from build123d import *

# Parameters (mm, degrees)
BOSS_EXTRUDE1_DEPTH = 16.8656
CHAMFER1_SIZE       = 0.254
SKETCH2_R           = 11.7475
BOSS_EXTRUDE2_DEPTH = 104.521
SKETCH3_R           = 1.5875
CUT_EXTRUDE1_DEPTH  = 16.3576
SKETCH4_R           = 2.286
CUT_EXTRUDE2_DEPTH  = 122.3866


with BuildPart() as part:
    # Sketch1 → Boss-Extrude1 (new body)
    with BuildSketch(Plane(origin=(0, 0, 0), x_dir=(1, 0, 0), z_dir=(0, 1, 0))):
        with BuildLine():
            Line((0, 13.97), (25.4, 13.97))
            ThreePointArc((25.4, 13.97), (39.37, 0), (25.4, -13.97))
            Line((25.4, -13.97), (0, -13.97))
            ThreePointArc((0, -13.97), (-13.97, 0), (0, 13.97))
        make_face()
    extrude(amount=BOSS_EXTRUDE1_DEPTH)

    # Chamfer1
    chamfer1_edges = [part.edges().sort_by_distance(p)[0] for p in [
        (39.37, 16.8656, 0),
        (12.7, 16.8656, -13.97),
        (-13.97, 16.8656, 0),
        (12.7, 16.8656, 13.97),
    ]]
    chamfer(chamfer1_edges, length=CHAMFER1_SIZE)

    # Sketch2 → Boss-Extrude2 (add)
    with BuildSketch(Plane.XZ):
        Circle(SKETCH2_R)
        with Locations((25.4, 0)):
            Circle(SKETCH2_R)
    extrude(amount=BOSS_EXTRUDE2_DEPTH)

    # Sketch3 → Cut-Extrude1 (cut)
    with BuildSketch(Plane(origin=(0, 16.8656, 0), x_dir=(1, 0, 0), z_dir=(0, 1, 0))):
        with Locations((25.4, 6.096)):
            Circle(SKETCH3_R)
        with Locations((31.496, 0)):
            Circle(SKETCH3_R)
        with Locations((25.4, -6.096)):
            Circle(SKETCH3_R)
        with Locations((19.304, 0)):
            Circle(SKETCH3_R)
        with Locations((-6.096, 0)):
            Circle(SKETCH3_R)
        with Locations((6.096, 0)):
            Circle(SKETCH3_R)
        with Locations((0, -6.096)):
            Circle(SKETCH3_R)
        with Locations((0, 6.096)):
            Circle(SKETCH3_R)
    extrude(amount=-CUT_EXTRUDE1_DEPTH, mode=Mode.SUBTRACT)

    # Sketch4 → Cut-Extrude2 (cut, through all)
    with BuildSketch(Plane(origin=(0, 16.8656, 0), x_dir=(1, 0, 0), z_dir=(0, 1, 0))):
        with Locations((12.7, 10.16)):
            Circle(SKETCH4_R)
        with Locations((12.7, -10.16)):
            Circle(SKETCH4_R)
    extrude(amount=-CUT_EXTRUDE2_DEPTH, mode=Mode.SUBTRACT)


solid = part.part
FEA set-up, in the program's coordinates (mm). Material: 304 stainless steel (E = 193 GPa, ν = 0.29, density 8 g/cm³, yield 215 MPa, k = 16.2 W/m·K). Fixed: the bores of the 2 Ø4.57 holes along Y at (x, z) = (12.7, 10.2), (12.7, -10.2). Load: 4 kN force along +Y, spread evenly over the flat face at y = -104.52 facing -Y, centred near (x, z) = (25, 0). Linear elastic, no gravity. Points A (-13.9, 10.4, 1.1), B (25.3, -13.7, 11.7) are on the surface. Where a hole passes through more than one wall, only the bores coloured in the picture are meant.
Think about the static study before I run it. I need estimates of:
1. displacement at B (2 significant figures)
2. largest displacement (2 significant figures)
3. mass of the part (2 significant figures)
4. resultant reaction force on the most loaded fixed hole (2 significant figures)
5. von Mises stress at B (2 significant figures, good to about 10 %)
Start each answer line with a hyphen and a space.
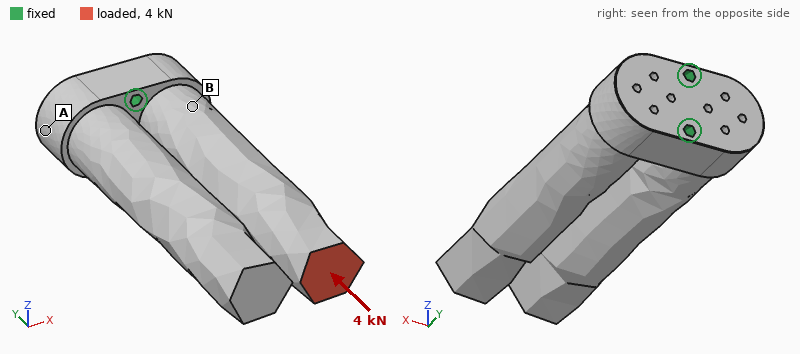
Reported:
- 5.9 µm
- 27 µm
- 890 g
- 2.0 kN
- 8.6 MPa
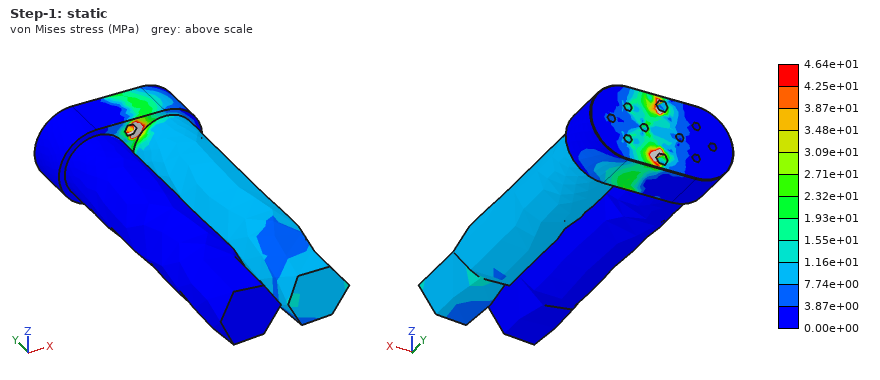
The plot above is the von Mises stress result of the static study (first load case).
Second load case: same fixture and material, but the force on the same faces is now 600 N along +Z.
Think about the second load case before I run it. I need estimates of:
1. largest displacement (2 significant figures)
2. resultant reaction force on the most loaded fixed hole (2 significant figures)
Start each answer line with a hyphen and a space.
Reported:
- 0.11 mm
- 2.7 kN
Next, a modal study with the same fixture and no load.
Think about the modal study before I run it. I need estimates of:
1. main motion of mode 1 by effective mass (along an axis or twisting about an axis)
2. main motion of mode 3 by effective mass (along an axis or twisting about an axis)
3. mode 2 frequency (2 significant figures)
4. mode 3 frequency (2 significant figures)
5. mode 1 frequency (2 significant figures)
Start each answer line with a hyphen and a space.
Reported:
- along X
- along Z
- 1100 Hz
- 1200 Hz
- 1000 Hz
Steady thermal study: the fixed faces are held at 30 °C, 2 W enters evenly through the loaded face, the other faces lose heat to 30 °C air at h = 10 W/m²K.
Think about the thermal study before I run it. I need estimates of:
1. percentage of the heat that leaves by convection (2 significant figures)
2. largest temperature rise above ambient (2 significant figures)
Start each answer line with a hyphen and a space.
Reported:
- 47 %
- 23 K
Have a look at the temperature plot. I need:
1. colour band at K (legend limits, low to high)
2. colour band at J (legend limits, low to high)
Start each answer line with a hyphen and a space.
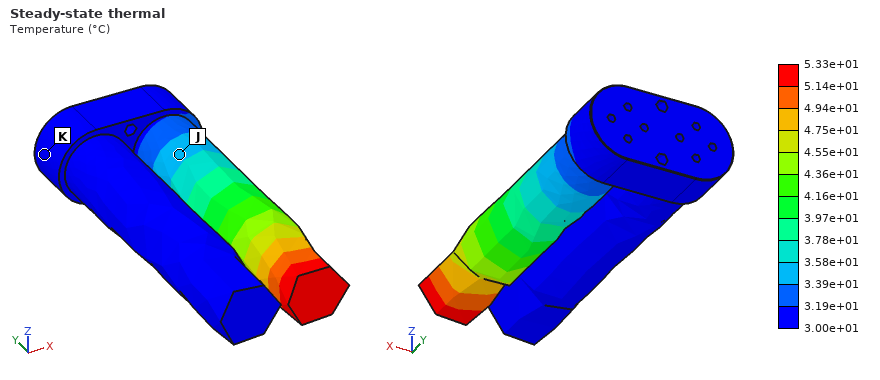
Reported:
- 3.00e+01 to 3.19e+01 °C
- 3.39e+01 to 3.58e+01 °C
